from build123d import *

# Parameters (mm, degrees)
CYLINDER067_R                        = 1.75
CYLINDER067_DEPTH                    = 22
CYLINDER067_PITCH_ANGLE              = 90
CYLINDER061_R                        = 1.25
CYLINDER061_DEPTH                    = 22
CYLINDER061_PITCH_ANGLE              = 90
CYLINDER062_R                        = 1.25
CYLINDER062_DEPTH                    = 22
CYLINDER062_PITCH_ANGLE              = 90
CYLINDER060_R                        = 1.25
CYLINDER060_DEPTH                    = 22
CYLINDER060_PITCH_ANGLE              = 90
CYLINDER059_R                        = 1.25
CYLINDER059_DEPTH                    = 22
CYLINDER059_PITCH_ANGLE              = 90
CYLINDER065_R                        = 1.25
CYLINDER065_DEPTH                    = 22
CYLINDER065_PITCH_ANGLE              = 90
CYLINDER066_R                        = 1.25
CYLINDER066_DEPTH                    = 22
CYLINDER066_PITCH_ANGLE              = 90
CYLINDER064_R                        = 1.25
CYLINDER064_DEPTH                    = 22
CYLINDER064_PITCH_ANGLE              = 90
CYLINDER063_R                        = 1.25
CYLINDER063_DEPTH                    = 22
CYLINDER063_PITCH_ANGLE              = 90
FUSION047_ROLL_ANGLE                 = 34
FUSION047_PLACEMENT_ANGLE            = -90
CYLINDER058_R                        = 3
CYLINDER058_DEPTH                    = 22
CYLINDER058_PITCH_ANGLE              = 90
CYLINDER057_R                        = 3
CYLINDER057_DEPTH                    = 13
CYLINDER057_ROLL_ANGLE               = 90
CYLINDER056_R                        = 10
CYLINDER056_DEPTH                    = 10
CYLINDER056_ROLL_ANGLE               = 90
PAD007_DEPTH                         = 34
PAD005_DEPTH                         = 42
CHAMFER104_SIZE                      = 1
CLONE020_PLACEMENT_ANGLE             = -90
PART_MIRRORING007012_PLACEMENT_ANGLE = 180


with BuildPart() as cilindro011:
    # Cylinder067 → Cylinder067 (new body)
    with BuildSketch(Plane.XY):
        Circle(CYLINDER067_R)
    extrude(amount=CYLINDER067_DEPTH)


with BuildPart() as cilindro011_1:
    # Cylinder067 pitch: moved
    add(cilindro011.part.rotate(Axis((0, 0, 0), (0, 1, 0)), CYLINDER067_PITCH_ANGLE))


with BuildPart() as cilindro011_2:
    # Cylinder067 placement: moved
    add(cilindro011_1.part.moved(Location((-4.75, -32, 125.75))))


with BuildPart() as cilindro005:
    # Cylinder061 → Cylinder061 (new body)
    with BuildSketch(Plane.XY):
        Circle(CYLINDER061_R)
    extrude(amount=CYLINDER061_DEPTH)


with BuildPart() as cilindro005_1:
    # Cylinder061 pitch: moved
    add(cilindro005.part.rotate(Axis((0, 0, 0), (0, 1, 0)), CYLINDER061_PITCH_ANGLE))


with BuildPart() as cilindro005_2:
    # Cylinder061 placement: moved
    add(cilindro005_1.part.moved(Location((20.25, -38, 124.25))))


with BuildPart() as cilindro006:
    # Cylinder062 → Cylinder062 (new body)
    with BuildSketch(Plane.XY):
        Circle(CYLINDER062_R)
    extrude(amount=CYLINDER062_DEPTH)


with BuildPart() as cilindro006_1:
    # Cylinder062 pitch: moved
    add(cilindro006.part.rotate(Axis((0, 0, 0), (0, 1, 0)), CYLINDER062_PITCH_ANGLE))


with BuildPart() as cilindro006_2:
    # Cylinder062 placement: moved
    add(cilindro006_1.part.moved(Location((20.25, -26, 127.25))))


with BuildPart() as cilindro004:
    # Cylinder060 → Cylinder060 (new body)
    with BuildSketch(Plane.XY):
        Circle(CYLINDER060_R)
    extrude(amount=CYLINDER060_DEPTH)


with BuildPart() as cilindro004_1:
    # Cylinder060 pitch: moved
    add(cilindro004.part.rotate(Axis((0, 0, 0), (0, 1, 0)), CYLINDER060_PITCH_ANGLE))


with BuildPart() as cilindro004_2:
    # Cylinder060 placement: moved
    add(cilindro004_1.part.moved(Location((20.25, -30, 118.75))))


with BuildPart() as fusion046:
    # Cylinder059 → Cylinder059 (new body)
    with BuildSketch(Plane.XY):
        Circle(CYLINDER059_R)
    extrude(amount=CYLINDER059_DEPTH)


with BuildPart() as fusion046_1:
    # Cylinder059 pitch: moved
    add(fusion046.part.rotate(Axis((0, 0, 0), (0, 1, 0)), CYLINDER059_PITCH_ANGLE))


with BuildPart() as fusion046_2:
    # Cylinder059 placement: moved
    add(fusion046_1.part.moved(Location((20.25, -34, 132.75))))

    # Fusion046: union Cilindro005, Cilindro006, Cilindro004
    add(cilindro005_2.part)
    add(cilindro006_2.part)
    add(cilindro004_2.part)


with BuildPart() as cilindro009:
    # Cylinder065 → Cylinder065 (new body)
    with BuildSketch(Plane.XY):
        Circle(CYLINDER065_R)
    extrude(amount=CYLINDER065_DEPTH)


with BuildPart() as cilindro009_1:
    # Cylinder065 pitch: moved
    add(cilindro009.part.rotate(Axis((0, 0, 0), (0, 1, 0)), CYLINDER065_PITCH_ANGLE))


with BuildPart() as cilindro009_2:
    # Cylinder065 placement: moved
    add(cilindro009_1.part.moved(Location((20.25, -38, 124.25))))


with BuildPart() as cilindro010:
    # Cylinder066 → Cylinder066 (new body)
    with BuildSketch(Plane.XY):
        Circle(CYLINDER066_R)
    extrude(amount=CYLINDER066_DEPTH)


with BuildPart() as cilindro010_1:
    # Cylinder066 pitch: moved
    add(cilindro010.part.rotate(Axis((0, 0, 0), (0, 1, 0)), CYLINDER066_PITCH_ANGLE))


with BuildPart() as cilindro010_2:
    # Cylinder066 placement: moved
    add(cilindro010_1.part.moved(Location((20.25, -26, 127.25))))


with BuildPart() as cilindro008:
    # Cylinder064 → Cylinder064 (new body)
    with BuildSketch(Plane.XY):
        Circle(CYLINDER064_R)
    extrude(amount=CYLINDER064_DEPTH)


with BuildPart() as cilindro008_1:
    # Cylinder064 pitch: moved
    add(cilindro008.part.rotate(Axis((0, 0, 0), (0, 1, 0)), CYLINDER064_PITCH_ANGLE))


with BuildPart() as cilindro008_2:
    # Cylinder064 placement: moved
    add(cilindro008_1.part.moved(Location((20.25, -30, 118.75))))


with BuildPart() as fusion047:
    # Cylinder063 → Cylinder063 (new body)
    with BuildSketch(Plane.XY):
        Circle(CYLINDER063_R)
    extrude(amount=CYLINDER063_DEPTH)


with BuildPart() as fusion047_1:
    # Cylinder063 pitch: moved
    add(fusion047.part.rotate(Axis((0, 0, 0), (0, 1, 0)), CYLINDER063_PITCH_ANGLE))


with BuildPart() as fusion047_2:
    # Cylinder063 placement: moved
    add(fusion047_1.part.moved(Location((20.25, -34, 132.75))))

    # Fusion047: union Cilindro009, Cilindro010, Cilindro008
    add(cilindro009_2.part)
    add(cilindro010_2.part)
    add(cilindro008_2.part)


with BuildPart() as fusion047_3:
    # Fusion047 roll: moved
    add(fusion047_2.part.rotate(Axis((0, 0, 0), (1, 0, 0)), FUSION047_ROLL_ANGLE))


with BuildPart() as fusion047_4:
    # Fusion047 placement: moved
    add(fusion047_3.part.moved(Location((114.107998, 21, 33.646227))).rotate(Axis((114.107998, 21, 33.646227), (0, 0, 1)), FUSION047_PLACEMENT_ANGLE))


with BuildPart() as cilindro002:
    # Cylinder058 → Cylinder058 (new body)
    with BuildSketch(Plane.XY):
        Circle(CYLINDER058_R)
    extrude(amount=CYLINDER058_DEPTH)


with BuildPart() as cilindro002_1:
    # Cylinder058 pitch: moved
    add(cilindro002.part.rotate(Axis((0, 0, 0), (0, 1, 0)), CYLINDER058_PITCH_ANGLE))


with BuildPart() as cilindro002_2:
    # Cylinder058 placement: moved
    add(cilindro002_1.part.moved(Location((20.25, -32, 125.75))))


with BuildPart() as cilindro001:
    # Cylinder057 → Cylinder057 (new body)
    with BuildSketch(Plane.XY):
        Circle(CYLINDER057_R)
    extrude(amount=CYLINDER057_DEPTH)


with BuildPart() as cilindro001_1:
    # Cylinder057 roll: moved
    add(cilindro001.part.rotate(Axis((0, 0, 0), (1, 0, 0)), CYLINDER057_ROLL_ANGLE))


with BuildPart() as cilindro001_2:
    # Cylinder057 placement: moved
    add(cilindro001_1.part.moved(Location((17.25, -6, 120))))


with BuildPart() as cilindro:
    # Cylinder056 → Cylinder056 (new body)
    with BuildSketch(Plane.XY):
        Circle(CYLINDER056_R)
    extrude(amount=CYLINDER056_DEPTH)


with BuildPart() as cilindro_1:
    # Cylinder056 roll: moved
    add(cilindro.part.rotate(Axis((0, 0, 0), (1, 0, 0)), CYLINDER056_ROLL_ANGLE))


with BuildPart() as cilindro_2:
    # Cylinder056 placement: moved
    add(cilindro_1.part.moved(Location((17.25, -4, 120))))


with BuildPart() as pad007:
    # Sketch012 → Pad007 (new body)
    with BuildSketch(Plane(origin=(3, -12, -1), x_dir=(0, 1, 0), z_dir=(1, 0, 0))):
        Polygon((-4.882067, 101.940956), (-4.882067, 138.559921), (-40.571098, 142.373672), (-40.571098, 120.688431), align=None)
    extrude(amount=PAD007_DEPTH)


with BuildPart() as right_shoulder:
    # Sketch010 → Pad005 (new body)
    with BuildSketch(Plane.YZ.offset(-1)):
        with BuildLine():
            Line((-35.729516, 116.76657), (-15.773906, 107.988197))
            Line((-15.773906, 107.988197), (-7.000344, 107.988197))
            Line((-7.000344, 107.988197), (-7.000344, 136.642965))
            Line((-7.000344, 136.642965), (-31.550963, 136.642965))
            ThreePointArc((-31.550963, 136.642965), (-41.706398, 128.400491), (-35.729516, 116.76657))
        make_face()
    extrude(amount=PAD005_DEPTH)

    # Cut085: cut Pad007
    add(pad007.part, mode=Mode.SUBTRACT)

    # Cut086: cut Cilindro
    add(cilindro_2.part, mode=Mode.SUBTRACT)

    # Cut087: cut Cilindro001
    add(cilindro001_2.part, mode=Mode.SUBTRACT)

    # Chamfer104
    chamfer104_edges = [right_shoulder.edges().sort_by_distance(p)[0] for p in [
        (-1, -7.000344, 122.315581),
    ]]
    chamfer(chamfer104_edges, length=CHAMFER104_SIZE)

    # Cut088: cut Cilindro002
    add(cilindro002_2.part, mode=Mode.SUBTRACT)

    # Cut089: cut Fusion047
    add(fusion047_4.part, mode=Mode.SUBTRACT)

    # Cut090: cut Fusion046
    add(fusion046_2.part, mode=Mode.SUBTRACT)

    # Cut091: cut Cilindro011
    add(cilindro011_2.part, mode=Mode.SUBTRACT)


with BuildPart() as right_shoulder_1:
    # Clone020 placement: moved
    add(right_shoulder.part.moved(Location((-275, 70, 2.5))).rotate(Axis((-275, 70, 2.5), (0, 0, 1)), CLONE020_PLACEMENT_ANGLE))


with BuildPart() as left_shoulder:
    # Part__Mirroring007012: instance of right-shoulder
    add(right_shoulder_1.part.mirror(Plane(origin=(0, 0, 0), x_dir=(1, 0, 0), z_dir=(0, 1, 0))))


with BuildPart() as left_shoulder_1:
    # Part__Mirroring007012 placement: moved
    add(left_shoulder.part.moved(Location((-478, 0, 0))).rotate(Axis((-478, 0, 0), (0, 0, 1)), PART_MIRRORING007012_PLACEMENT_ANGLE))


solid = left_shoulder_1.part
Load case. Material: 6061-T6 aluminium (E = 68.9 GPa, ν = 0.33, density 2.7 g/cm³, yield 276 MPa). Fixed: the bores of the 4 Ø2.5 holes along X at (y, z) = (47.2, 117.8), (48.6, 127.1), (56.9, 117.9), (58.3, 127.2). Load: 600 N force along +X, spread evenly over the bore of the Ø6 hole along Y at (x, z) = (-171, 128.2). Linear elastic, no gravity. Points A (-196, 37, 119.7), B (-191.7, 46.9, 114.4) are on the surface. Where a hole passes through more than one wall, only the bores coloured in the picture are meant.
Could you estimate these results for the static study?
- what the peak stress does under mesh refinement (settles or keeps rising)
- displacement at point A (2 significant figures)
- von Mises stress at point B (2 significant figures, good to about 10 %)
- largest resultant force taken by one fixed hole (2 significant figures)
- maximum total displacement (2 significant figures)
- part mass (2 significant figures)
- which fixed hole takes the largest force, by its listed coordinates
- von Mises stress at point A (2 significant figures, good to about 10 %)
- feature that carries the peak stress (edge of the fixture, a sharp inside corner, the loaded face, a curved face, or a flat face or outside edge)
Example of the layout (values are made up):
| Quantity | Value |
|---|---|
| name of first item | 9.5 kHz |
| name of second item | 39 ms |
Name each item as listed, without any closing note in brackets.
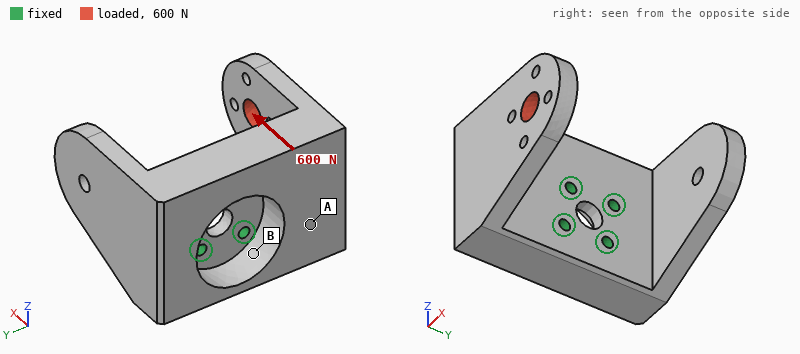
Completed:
| Quantity | Value |
|---|---|
| what the peak stress does under mesh refinement | keeps rising |
| displacement at point A | 30 µm |
| von Mises stress at point B | 33 MPa |
| largest resultant force taken by one fixed hole | 800 N |
| maximum total displacement | 88 µm |
| part mass | 37 g |
| which fixed hole takes the largest force, by its listed coordinates | (48.6, 127.1) |
| von Mises stress at point A | 15 MPa |
| feature that carries the peak stress | edge of the fixture |
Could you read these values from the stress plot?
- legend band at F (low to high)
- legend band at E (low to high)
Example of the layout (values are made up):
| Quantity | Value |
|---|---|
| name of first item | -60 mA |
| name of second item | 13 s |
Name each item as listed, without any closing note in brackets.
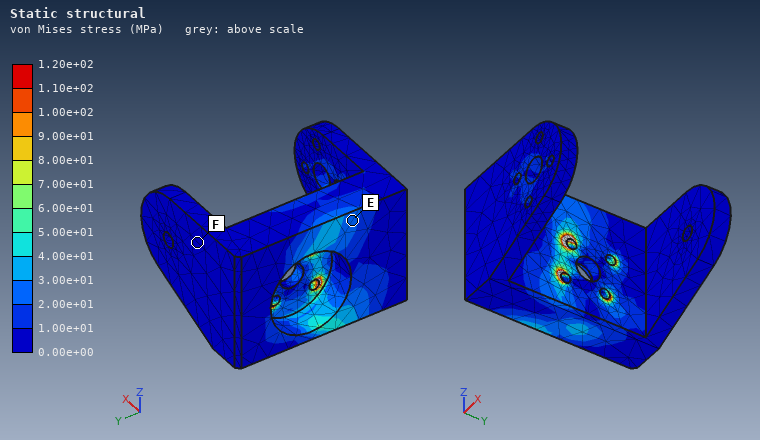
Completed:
| Quantity | Value |
|---|---|
| legend band at F | 0.00e+00 to 1.00e+01 MPa |
| legend band at E | 2.00e+01 to 3.00e+01 MPa |
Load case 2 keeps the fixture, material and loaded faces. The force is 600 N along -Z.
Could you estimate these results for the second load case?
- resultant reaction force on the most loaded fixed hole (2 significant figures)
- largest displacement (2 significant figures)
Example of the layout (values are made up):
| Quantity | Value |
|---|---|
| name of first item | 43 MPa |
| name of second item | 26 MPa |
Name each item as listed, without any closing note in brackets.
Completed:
| Quantity | Value |
|---|---|
| resultant reaction force on the most loaded fixed hole | 770 N |
| largest displacement | 85 µm |
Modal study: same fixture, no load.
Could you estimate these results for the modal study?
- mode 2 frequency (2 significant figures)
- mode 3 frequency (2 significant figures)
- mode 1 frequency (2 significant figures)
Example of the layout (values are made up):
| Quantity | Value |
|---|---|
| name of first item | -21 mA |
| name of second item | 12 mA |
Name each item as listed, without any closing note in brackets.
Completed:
| Quantity | Value |
|---|---|
| mode 2 frequency | 5000 Hz |
| mode 3 frequency | 6300 Hz |
| mode 1 frequency | 4000 Hz |
